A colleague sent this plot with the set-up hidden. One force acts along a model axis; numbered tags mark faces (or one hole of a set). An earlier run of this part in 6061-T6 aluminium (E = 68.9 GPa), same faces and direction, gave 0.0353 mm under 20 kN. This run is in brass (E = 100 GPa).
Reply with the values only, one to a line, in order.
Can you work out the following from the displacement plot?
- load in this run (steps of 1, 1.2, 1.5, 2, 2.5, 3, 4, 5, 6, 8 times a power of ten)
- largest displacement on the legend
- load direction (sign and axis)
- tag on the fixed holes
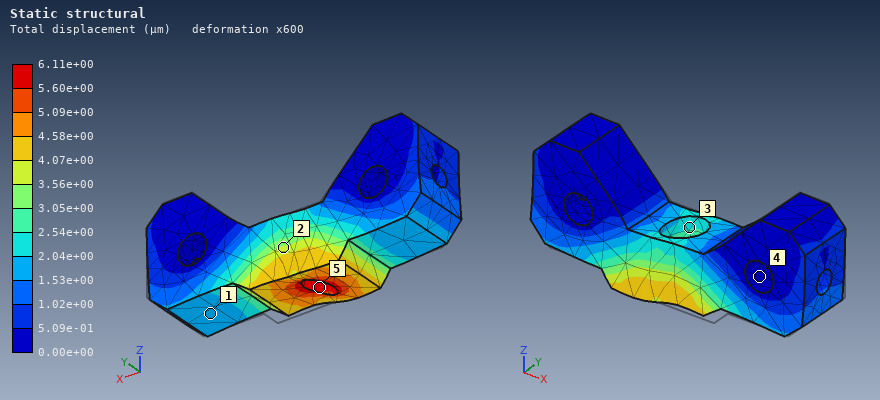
5 kN
6.11e+00 µm
-X
4
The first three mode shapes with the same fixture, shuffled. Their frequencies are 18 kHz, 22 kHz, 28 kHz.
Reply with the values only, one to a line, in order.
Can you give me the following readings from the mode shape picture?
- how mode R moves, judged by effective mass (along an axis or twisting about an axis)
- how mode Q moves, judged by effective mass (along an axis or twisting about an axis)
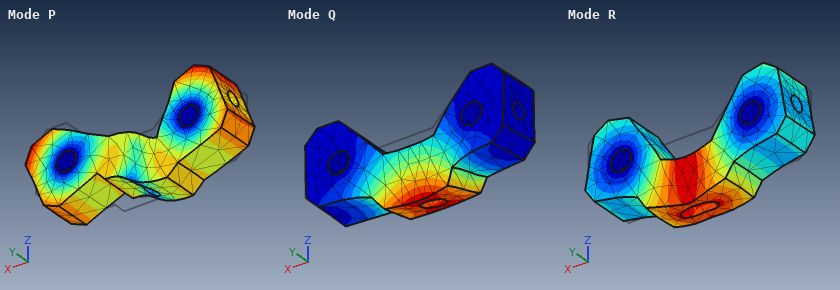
along Z
along Y
